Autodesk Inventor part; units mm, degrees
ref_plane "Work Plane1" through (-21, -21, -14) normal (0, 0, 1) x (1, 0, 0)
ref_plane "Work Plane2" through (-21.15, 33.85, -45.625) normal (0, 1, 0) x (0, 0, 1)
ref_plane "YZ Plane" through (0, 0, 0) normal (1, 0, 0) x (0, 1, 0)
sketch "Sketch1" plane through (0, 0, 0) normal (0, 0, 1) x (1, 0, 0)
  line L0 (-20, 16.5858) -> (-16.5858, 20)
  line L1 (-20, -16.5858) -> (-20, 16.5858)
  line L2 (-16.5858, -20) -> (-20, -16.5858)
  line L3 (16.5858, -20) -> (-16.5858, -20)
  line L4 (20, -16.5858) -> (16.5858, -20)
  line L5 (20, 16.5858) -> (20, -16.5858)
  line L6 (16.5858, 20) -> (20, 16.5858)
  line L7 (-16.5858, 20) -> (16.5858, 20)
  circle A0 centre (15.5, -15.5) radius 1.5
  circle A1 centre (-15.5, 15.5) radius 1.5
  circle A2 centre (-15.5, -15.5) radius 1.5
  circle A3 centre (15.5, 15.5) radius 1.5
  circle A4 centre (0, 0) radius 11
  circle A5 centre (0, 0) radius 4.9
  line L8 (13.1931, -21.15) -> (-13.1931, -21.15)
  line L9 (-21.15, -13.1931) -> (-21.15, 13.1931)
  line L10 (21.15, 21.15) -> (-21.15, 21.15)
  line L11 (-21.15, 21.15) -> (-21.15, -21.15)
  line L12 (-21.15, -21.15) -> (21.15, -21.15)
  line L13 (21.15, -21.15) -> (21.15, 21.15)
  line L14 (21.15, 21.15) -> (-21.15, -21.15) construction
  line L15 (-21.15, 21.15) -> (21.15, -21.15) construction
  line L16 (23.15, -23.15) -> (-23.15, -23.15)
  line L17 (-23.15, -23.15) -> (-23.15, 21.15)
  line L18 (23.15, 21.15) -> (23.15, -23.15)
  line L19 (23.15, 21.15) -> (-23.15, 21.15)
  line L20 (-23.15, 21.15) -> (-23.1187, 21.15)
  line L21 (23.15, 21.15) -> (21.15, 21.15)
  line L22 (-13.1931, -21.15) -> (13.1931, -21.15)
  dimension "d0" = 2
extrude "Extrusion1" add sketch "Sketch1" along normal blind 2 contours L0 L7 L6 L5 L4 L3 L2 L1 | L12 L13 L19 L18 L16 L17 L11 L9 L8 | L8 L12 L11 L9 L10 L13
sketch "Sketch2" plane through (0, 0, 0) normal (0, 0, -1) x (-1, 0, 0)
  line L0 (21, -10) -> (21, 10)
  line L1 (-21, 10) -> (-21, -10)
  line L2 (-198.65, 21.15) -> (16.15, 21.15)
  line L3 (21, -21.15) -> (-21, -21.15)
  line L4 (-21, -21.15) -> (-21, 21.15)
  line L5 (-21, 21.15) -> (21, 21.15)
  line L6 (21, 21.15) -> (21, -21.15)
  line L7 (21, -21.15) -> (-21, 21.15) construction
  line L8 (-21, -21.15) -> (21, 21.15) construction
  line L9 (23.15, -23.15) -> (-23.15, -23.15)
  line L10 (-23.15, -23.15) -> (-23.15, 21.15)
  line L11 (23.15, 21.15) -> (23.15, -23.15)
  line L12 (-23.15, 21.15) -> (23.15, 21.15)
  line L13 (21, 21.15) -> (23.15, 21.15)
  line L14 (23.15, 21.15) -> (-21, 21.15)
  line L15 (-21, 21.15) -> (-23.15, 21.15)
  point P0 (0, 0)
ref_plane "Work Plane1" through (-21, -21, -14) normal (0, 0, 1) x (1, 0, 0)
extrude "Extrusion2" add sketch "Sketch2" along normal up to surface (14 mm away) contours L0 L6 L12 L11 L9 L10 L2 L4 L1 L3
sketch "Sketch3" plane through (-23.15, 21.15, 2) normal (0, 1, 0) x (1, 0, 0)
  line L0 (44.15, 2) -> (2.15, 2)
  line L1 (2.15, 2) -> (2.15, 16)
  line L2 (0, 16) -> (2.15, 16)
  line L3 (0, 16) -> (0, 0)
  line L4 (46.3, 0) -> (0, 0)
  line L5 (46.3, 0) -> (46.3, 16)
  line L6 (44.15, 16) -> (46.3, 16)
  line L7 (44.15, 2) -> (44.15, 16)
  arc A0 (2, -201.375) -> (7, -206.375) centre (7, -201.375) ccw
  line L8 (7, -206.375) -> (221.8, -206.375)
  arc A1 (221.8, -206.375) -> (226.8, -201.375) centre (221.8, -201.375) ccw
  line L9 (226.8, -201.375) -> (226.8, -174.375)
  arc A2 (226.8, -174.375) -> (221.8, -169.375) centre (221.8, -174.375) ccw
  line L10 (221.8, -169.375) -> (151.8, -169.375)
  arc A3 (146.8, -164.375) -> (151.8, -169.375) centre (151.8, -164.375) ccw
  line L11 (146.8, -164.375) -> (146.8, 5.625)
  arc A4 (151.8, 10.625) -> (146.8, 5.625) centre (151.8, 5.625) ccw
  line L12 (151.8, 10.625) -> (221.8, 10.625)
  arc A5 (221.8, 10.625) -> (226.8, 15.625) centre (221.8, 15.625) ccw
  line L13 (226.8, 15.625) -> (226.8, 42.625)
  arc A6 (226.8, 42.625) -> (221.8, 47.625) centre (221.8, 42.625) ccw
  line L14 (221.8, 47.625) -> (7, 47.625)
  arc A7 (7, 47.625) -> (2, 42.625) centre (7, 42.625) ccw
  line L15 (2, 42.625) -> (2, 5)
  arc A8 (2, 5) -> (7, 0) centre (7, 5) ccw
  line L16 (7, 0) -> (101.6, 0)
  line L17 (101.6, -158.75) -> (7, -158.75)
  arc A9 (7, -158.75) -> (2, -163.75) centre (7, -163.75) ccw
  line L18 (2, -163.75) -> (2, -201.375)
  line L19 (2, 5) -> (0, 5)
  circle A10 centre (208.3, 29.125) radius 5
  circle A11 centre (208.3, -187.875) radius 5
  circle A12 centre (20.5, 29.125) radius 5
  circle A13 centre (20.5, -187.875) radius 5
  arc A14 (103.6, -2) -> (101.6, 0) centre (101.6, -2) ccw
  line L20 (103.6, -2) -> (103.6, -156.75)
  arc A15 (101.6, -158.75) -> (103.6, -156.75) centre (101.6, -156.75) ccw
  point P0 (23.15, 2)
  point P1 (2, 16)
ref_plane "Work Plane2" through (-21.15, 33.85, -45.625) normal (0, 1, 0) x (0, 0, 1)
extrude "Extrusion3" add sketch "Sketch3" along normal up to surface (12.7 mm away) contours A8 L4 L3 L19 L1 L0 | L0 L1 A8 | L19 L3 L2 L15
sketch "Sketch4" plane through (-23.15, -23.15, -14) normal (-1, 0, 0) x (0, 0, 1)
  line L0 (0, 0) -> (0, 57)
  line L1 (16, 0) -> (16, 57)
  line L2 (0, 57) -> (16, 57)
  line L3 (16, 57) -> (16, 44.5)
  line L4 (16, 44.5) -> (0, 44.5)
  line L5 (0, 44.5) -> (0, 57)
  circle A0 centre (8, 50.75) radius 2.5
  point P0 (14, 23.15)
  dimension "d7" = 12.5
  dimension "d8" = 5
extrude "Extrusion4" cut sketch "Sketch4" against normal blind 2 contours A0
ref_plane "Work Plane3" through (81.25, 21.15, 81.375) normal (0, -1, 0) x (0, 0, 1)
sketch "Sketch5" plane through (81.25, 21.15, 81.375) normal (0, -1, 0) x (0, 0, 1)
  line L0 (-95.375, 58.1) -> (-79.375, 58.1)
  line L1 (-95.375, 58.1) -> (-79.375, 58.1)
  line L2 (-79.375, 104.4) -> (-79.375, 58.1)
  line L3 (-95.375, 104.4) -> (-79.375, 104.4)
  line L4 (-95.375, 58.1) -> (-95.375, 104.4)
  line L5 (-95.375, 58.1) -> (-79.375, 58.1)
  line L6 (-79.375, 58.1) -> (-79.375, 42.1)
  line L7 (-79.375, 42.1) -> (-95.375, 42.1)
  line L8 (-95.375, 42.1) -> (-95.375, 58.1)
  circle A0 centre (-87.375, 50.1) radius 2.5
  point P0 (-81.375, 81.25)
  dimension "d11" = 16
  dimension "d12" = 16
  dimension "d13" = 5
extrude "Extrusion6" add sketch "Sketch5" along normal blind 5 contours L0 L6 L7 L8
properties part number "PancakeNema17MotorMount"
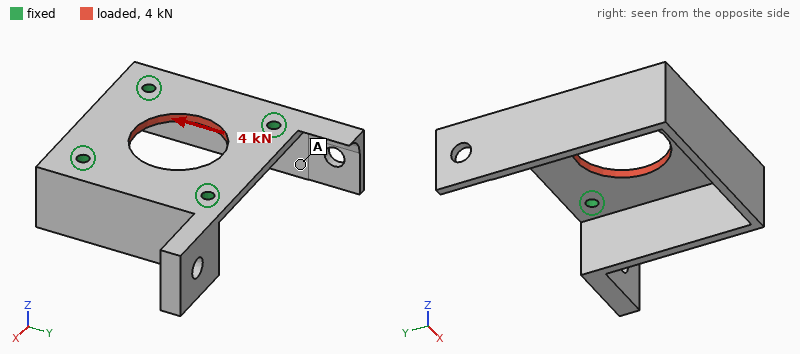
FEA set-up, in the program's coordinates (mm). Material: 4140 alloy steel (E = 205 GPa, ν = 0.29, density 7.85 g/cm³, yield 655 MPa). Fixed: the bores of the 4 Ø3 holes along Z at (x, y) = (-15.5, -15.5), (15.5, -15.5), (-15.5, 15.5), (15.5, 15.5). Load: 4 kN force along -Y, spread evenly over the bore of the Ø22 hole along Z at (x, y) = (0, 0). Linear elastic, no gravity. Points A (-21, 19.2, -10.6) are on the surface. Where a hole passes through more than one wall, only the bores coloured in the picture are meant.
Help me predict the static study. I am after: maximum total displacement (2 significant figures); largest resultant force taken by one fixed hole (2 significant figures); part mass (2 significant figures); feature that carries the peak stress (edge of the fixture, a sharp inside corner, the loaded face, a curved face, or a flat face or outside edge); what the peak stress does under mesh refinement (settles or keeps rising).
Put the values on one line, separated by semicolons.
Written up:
6.0 µm; 1.0 kN; 69 g; edge of the fixture; keeps rising
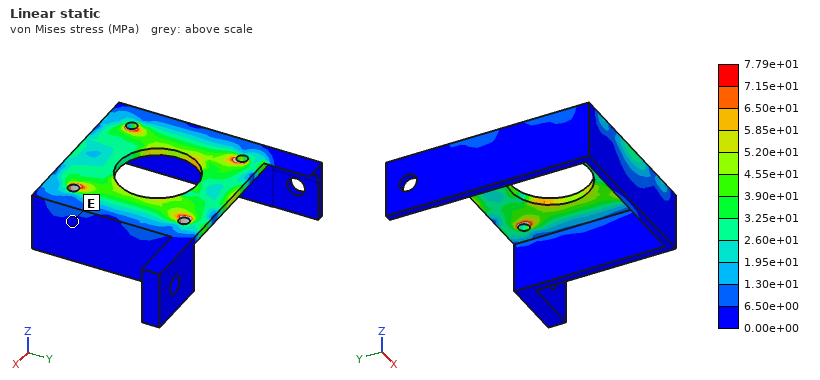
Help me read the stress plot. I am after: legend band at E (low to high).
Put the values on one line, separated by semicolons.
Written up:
0.00e+00 to 6.50e+00 MPa
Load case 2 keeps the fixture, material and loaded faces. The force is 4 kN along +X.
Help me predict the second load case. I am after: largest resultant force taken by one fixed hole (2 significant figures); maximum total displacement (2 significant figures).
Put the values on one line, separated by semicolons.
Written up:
1.0 kN; 5.0 µm
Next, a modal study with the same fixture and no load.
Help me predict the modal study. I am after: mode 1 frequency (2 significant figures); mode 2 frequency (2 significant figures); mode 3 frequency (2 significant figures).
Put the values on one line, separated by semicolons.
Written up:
2100 Hz; 3900 Hz; 5700 Hz
